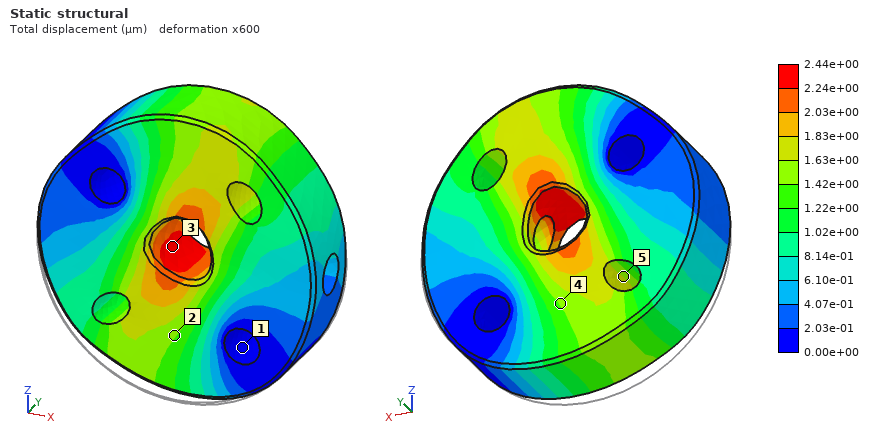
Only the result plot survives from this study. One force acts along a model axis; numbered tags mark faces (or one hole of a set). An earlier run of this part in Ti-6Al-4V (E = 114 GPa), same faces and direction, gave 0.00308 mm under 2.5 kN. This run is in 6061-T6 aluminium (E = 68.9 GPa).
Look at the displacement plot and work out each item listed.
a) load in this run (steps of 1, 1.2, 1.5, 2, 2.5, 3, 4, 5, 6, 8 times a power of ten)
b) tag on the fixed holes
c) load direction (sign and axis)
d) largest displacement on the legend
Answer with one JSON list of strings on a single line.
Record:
["1.2 kN", "1", "+Z", "2.44e+00 µm"]
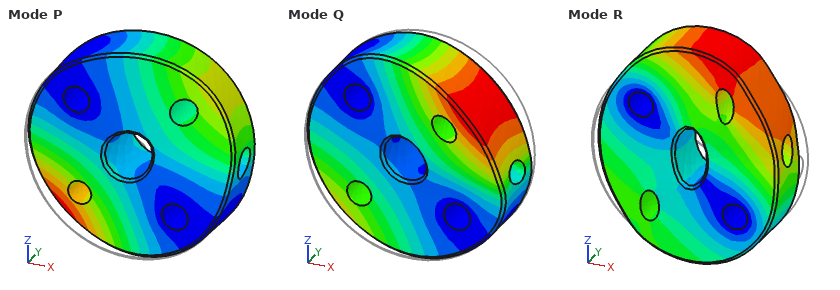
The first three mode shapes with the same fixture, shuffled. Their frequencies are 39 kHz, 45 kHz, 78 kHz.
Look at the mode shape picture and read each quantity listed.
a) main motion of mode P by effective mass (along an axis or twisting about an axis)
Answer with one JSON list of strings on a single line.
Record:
["along Y"]
